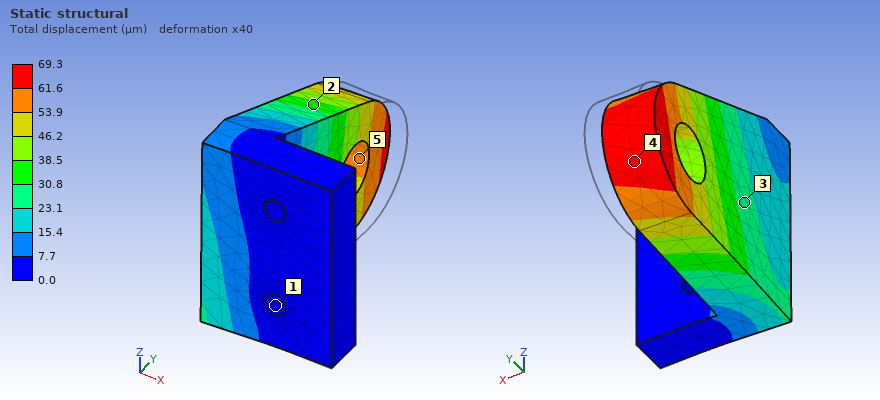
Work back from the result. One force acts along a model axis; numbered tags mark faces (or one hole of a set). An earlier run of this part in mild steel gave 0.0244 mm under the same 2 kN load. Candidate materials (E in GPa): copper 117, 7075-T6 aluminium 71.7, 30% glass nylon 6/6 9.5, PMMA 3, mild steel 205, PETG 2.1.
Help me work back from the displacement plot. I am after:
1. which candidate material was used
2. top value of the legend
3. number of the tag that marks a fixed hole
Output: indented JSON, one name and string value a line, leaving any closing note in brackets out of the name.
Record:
{
  "which candidate material was used": "7075-T6 aluminium",
  "top value of the legend": "69.3 µm",
  "number of the tag that marks a fixed hole": "1"
}
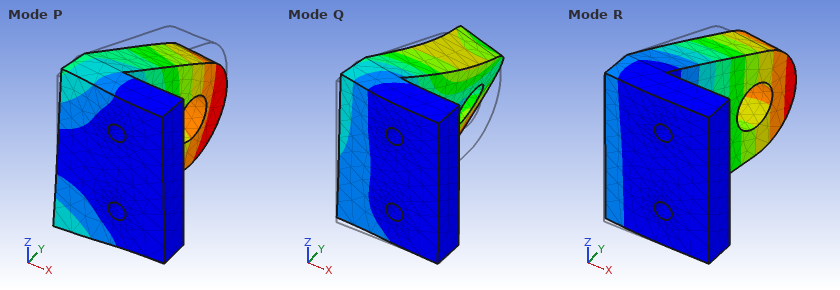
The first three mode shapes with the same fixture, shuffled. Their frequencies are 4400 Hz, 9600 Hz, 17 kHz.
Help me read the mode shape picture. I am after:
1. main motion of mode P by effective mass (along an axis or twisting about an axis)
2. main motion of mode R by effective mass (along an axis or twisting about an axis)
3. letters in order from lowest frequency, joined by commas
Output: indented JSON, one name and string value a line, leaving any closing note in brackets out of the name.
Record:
{
  "main motion of mode P by effective mass": "along Z",
  "main motion of mode R by effective mass": "along X",
  "letters in order from lowest frequency, joined by commas": "R, P, Q"
}
